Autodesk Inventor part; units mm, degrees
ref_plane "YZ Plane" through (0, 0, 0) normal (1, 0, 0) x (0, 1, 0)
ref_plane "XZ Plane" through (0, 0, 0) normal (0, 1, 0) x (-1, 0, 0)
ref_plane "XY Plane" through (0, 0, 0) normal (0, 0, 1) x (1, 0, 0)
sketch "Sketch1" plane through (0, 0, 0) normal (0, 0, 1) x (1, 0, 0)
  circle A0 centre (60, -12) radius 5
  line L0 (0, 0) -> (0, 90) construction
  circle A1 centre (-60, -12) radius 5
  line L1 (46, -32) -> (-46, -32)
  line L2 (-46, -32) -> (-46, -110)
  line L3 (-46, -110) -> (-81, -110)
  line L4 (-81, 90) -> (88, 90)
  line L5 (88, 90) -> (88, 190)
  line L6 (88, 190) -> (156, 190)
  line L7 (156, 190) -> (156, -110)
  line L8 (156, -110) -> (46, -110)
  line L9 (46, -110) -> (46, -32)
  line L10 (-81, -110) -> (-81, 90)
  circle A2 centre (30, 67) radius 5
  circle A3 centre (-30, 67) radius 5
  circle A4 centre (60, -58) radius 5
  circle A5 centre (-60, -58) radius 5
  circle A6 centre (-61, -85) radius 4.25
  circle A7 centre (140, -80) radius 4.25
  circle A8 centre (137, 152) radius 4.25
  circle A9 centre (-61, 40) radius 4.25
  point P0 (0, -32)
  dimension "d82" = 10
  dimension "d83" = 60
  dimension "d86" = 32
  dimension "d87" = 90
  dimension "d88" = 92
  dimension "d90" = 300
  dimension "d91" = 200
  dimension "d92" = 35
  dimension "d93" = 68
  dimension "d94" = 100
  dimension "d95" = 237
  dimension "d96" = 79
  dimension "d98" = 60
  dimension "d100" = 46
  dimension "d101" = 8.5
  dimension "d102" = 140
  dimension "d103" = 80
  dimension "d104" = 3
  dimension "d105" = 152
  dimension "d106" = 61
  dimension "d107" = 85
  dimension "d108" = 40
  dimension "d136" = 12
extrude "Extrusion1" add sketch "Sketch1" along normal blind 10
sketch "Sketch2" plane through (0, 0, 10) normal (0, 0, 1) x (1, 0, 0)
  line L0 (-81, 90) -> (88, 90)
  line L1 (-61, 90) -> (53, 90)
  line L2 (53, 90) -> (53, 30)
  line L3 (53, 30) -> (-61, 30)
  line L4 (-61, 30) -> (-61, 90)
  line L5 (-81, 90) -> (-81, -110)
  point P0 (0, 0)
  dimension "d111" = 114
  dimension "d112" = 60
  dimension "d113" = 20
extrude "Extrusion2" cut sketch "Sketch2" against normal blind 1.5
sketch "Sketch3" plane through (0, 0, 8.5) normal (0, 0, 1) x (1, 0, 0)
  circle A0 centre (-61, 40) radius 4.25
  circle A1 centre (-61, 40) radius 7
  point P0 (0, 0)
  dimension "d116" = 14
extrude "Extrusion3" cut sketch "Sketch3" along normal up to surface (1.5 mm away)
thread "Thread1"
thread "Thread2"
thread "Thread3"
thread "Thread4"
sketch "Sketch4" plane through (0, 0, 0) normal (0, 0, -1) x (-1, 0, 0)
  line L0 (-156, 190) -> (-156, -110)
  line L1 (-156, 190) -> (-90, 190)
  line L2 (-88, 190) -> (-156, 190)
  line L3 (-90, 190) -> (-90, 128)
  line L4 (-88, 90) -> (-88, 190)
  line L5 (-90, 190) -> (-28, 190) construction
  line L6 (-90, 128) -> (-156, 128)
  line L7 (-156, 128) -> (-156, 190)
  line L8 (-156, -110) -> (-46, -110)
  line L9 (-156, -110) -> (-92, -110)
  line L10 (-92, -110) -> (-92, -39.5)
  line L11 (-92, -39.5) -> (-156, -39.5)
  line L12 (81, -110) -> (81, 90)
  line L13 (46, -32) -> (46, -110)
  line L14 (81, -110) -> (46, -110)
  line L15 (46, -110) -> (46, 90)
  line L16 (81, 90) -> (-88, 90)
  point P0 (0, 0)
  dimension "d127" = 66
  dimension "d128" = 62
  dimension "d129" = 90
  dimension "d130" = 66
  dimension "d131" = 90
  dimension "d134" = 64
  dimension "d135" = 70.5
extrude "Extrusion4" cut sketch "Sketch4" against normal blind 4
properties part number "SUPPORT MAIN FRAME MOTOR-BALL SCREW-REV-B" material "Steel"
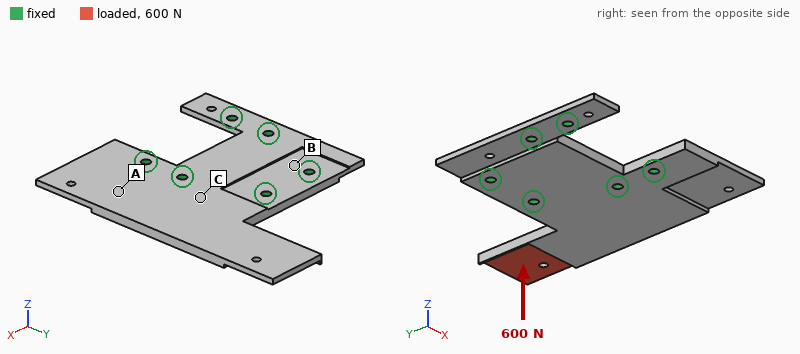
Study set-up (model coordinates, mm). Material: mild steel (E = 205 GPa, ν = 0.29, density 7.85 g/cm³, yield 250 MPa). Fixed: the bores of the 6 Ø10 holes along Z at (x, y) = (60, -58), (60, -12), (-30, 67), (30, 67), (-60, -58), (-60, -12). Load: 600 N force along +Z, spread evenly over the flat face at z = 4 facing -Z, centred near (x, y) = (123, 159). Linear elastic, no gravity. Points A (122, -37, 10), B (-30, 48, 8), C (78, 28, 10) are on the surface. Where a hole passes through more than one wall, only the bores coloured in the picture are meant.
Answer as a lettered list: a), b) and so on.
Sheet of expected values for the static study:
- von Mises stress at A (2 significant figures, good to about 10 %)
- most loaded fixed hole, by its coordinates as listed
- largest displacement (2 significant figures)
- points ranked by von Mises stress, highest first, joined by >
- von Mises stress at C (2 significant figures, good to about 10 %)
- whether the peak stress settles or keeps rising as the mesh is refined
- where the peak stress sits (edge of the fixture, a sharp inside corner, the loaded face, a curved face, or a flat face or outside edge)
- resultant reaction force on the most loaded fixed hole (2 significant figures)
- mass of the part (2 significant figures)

a) 11 MPa
b) (30, 67)
c) 0.65 mm
d) C > A > B
e) 25 MPa
f) keeps rising
g) edge of the fixture
h) 990 N
i) 3.1 kg
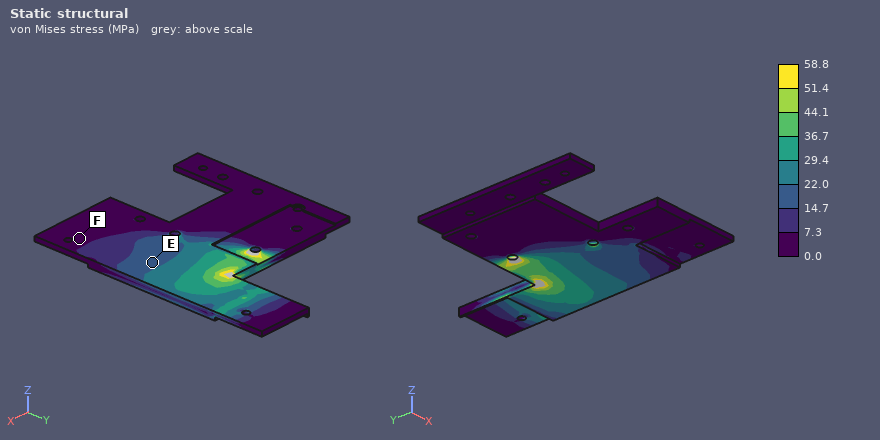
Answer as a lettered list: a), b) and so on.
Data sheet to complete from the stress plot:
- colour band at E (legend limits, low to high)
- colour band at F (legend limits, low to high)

a) 14.7 to 22.0 MPa
b) 0.0 to 7.3 MPa
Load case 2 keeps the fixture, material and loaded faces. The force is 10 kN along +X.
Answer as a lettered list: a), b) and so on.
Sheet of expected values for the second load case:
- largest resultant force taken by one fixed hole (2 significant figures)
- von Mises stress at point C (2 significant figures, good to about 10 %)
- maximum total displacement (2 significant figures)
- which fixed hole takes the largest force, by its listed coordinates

a) 13 kN
b) 13 MPa
c) 0.22 mm
d) (30, 67)
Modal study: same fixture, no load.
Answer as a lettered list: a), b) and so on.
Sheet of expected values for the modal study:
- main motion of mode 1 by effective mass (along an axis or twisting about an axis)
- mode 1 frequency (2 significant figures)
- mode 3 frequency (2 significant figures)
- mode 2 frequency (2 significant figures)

a) along Z
b) 340 Hz
c) 1100 Hz
d) 780 Hz
